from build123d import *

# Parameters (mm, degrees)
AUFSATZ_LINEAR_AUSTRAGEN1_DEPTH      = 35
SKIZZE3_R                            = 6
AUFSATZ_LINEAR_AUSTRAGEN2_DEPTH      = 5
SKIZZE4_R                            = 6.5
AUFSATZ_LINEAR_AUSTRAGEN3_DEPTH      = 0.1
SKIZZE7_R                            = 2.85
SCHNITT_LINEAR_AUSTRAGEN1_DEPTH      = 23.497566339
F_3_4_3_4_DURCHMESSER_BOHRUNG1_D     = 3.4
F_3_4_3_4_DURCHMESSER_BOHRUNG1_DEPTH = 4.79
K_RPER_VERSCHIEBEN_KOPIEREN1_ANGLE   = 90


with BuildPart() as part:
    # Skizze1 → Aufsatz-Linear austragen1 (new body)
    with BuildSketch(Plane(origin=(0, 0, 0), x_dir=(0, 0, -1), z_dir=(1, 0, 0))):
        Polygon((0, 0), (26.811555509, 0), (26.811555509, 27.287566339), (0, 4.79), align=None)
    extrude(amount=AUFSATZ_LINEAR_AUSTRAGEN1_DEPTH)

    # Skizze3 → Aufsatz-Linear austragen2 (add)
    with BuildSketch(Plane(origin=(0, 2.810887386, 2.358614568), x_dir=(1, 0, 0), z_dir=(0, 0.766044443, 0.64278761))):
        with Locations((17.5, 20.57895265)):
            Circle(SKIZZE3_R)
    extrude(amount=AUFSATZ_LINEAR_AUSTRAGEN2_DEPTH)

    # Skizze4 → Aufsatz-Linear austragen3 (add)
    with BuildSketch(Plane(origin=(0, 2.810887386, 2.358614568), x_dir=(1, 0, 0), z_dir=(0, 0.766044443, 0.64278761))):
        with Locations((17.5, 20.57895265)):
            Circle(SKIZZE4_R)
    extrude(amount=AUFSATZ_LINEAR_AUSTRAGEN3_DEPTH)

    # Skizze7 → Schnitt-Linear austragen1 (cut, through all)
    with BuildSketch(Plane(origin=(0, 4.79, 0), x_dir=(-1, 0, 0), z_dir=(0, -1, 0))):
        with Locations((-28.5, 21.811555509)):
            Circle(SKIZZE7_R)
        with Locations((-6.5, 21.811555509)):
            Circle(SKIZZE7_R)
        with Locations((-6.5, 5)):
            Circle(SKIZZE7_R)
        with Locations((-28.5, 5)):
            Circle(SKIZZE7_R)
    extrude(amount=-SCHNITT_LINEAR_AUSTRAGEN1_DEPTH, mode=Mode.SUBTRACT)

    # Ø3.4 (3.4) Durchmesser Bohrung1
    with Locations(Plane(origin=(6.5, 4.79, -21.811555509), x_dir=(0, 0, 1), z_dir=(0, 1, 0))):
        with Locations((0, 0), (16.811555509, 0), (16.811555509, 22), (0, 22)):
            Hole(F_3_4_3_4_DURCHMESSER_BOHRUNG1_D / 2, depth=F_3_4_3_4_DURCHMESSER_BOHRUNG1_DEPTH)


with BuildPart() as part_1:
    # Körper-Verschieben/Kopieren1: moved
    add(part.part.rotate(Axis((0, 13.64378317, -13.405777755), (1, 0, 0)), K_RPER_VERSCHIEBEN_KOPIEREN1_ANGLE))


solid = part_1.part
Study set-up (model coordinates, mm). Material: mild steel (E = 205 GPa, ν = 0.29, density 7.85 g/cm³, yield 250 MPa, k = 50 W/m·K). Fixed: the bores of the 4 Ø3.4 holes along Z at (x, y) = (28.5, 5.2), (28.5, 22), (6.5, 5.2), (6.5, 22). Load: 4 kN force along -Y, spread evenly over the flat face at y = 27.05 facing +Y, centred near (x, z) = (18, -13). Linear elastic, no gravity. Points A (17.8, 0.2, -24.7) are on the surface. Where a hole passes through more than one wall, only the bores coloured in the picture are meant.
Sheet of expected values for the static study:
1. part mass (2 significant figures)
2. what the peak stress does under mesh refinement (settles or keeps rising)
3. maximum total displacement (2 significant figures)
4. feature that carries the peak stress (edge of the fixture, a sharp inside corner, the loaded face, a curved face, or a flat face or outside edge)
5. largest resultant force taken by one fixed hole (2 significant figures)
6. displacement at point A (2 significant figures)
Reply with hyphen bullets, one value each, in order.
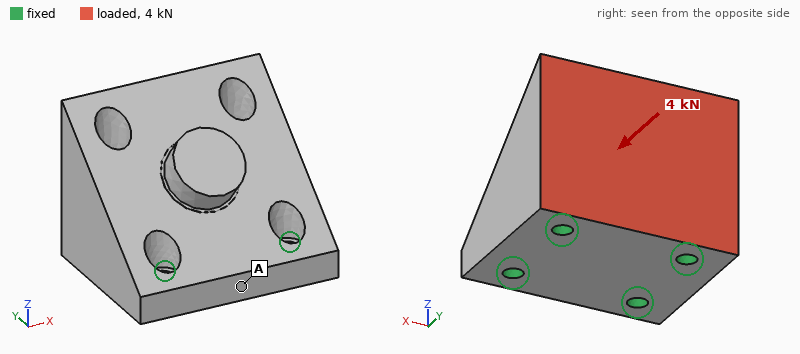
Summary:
- 110 g
- keeps rising
- 8.6 µm
- edge of the fixture
- 1.6 kN
- 1.6 µm
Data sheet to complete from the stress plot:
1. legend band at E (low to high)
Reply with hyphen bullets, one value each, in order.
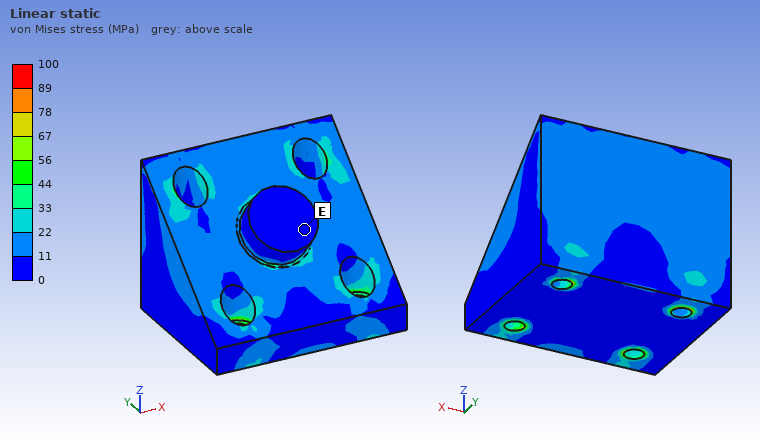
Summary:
- 0 to 11 MPa
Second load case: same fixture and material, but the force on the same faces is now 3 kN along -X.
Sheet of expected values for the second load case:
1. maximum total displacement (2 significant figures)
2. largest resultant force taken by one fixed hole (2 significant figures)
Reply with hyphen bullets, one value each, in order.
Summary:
- 4.6 µm
- 1.6 kN
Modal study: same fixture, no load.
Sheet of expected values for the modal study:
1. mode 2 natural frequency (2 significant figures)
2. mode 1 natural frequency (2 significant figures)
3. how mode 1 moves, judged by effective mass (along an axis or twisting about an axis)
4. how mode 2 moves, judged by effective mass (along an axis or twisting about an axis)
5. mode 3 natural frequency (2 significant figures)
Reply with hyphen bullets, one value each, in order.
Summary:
- 23 kHz
- 21 kHz
- along Y
- along X
- 34 kHz
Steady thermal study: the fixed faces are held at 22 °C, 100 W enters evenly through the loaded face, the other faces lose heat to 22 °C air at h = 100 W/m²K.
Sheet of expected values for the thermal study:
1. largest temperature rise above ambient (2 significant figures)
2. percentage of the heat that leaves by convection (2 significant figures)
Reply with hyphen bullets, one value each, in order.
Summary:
- 85 K
- 12 %
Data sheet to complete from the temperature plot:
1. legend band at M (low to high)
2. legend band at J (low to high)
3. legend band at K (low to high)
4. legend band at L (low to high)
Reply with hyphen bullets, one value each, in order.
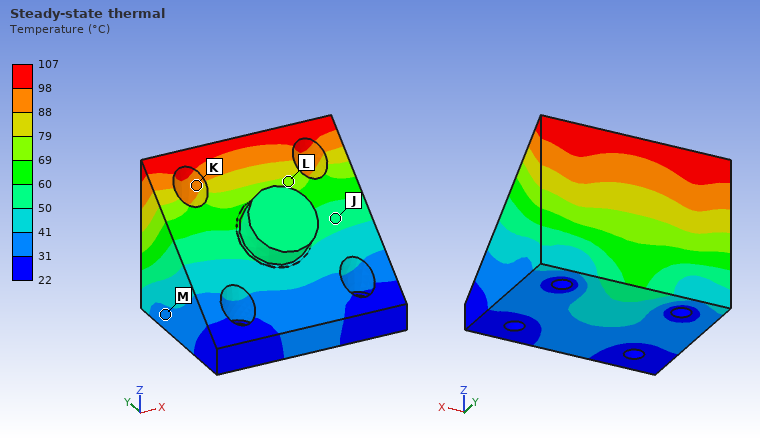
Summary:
- 31 to 41 °C
- 50 to 60 °C
- 88 to 98 °C
- 69 to 79 °C
